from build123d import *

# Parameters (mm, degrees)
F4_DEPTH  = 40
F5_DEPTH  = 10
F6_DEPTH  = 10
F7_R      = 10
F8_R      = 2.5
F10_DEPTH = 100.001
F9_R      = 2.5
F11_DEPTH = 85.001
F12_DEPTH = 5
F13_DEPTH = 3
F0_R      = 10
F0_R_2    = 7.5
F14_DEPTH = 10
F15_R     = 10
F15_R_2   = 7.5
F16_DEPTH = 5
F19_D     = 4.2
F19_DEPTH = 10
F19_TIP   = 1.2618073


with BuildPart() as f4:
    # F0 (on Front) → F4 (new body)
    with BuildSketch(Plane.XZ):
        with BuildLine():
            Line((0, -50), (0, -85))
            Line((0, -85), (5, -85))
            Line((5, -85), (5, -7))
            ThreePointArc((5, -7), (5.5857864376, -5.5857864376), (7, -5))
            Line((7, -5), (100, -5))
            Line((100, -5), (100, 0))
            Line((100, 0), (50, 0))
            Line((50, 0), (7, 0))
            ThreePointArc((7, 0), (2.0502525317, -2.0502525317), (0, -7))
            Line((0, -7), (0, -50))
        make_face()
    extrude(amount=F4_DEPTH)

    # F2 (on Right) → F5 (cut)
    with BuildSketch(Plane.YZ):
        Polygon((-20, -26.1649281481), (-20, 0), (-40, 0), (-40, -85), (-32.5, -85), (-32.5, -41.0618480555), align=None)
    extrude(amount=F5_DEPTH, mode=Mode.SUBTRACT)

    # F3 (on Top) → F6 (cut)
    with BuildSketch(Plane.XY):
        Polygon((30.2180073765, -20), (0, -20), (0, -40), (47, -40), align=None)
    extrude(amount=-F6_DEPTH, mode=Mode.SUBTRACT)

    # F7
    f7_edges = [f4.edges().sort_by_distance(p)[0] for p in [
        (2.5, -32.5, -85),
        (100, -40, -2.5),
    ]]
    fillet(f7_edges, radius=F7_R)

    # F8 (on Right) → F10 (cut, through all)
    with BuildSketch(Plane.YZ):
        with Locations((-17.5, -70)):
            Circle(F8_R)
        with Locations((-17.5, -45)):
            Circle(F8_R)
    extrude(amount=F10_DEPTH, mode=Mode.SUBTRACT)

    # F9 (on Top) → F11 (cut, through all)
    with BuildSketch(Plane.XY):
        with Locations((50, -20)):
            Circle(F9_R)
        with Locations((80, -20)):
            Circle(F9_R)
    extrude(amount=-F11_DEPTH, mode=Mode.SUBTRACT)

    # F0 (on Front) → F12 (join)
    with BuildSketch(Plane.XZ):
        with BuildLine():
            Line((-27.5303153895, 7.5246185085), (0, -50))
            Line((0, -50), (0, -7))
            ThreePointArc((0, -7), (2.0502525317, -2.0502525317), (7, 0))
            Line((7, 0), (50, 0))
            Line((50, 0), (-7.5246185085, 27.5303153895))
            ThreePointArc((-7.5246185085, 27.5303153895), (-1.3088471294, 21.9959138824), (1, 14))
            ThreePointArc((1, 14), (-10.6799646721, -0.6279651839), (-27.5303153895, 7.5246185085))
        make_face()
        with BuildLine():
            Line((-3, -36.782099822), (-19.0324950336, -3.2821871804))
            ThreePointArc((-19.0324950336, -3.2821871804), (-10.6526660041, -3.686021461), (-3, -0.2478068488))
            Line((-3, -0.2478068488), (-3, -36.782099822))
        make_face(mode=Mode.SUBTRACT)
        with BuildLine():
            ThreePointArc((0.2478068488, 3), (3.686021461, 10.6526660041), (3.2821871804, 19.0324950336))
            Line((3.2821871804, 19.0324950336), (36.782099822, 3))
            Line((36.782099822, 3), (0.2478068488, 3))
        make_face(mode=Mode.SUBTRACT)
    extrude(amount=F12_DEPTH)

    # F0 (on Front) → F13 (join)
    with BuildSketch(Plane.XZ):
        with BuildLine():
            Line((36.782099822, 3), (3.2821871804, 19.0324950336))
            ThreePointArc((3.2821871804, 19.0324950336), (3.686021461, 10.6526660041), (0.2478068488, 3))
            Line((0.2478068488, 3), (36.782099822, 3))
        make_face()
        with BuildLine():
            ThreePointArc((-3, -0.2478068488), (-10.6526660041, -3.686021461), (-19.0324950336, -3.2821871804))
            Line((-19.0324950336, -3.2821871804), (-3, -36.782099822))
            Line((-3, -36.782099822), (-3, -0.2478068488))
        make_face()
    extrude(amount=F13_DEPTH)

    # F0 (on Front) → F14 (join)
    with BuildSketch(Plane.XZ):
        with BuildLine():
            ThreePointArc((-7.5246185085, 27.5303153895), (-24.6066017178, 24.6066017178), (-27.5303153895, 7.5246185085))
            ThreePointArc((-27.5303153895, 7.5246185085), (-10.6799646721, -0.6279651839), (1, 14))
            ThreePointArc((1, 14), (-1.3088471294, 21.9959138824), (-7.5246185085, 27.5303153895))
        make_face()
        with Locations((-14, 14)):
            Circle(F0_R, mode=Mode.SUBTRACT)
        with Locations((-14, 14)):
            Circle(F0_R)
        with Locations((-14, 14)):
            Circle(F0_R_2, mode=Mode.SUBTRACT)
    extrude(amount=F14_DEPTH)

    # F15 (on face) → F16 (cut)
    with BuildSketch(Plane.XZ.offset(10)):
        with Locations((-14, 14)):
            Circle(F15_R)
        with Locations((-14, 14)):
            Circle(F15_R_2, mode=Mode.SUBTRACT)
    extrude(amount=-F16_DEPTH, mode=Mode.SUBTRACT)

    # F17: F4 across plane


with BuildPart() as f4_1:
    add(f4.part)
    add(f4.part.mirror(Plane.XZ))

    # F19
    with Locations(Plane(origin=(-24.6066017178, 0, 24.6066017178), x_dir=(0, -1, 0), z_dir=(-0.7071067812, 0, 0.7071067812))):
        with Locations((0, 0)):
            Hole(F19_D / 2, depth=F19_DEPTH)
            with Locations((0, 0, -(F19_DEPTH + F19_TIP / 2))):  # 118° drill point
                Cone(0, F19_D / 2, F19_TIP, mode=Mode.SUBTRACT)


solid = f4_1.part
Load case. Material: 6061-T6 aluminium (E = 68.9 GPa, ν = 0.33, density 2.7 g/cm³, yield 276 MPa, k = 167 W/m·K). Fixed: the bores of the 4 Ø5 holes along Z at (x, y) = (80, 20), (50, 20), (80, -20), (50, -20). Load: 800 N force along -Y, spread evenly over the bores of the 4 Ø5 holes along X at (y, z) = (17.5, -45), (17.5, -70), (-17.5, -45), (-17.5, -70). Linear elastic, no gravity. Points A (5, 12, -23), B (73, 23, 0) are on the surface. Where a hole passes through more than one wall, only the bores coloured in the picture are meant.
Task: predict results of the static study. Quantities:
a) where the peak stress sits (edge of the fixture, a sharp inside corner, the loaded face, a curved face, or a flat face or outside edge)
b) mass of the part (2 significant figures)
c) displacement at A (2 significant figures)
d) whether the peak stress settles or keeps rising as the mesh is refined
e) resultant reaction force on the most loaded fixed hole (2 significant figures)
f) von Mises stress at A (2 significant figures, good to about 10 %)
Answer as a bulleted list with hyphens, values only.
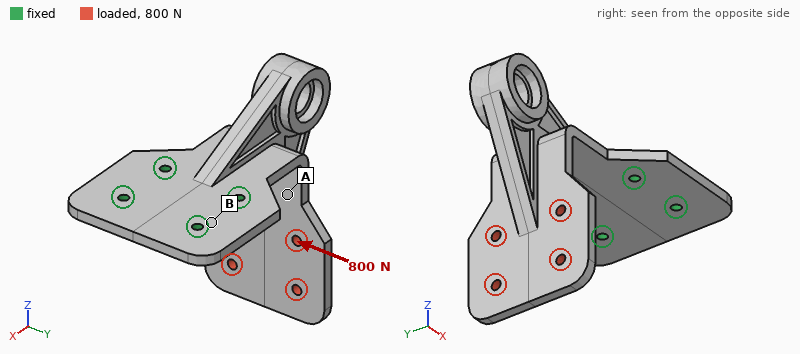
- edge of the fixture
- 200 g
- 0.46 mm
- keeps rising
- 1.5 kN
- 22 MPa
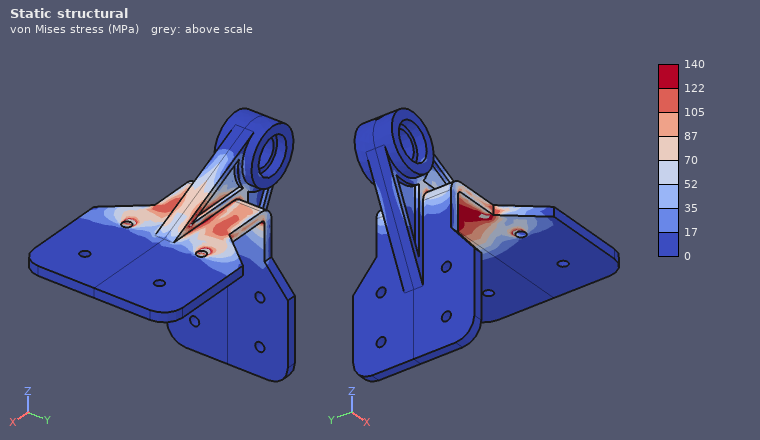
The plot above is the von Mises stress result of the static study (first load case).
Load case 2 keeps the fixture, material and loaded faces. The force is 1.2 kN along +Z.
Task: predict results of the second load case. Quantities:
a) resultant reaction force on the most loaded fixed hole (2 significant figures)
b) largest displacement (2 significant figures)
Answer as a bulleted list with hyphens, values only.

- 1.0 kN
- 1.6 mm
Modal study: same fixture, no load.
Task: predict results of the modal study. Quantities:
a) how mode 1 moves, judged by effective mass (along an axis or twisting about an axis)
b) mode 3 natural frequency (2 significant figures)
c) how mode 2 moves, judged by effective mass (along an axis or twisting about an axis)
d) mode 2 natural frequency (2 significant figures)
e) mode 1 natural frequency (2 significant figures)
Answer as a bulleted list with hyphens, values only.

- along Z
- 1500 Hz
- along Y
- 570 Hz
- 410 Hz
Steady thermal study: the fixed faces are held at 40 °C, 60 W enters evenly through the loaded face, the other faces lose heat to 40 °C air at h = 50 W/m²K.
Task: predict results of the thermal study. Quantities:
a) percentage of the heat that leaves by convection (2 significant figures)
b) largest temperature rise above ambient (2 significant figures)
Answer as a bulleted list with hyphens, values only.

- 64 %
- 68 K
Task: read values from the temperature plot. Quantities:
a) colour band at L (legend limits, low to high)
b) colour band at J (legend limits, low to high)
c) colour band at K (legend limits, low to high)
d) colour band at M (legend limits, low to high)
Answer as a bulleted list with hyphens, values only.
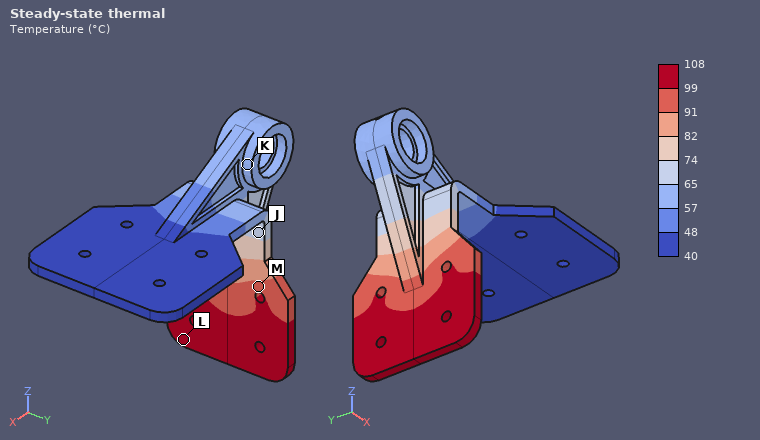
- 99 to 108 °C
- 65 to 74 °C
- 57 to 65 °C
- 91 to 99 °C
